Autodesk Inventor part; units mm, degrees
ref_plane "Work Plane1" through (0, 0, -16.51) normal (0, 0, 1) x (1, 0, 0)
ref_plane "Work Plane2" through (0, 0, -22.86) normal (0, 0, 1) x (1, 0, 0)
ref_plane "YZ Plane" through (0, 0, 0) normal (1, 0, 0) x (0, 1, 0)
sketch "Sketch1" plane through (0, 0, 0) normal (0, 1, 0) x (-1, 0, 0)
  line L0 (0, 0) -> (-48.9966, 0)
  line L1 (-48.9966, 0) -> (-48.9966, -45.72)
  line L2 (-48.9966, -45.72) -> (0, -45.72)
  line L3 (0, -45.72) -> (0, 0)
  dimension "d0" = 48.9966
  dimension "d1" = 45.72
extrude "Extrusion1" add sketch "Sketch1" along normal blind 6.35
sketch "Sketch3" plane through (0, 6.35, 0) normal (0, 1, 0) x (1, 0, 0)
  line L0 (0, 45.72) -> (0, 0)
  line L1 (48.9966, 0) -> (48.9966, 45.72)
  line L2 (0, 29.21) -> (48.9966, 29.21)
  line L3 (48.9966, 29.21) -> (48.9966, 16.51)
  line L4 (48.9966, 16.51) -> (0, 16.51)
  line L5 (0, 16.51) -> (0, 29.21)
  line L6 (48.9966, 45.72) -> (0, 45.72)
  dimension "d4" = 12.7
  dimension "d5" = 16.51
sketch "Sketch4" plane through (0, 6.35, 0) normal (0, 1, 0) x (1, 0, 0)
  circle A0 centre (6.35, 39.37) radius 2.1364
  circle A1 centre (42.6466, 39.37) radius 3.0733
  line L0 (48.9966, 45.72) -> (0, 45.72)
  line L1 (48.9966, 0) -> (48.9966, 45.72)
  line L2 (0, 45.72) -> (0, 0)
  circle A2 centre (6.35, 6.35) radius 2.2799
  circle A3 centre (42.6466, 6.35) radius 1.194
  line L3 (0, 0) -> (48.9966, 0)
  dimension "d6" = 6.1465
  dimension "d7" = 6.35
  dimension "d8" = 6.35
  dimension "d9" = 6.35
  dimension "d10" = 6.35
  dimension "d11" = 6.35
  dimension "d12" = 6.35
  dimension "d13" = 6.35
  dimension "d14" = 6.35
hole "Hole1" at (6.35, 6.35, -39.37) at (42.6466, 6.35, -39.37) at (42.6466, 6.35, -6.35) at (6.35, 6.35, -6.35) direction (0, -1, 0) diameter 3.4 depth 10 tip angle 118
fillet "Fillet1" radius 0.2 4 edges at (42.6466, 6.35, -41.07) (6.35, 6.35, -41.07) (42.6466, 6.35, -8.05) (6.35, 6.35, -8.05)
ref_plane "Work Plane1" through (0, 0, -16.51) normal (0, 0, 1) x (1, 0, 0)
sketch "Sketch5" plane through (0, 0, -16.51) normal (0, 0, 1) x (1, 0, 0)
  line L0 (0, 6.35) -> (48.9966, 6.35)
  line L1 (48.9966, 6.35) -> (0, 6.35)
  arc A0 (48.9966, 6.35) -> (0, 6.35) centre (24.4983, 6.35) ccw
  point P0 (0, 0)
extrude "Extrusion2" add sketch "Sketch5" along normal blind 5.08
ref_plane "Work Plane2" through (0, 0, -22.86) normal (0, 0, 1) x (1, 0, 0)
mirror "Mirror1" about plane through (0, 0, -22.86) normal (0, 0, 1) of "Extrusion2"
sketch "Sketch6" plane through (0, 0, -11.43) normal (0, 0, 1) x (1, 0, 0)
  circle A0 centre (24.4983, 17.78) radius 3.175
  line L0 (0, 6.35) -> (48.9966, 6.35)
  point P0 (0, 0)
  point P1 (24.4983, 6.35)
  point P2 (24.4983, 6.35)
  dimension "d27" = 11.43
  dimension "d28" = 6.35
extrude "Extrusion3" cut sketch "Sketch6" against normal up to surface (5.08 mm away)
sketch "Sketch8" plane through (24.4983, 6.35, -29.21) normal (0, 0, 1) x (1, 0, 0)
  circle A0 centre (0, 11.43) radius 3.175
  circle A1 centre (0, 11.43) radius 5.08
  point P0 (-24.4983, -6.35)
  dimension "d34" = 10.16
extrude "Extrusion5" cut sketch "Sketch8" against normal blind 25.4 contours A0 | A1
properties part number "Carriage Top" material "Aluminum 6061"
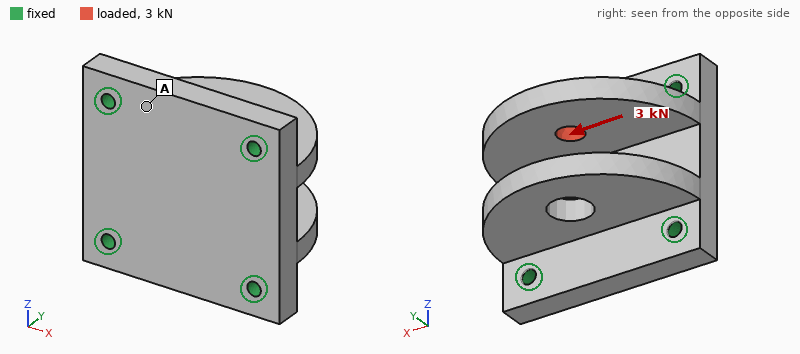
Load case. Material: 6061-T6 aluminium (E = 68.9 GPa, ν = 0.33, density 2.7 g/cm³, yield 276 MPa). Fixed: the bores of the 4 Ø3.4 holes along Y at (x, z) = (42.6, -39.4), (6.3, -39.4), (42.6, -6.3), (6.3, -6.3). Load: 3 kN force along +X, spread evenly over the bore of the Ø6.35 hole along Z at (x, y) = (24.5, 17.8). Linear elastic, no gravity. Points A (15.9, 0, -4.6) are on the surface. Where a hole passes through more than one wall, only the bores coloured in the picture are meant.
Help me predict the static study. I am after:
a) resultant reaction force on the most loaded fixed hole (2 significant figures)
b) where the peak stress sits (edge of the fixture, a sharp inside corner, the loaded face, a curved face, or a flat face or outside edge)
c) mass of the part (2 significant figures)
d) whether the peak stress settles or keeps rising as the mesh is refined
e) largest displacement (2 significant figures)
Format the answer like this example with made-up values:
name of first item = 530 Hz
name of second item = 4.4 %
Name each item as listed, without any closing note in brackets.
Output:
resultant reaction force on the most loaded fixed hole = 1.5 kN
where the peak stress sits = edge of the fixture
mass of the part = 62 g
whether the peak stress settles or keeps rising as the mesh is refined = keeps rising
largest displacement = 21 µm
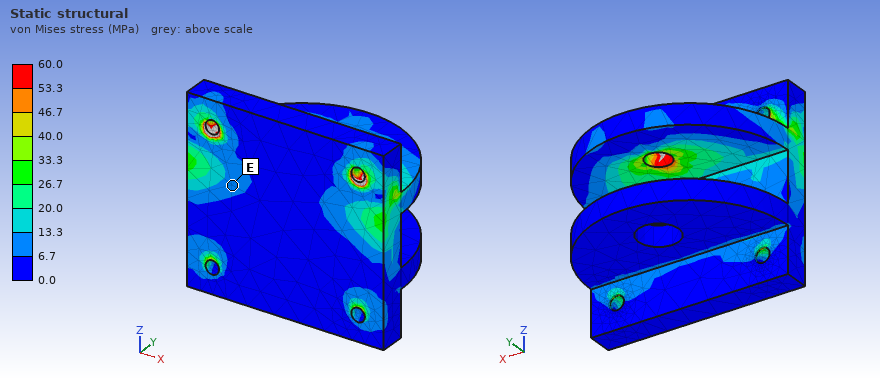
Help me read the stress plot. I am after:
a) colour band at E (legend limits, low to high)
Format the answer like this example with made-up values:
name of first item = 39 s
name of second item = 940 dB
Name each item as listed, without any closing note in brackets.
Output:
colour band at E = 6.7 to 13.3 MPa
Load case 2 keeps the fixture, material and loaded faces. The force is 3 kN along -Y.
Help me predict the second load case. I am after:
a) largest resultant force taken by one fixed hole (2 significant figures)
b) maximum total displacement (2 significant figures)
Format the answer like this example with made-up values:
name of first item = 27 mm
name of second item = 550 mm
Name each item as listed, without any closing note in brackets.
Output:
largest resultant force taken by one fixed hole = 1.2 kN
maximum total displacement = 19 µm
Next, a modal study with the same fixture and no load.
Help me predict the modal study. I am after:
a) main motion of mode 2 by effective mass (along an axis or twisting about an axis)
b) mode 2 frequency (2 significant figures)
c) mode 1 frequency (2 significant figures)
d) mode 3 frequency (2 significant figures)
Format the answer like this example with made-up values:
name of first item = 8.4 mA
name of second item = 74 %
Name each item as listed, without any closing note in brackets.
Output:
main motion of mode 2 by effective mass = along Z
mode 2 frequency = 7400 Hz
mode 1 frequency = 6600 Hz
mode 3 frequency = 13 kHz
